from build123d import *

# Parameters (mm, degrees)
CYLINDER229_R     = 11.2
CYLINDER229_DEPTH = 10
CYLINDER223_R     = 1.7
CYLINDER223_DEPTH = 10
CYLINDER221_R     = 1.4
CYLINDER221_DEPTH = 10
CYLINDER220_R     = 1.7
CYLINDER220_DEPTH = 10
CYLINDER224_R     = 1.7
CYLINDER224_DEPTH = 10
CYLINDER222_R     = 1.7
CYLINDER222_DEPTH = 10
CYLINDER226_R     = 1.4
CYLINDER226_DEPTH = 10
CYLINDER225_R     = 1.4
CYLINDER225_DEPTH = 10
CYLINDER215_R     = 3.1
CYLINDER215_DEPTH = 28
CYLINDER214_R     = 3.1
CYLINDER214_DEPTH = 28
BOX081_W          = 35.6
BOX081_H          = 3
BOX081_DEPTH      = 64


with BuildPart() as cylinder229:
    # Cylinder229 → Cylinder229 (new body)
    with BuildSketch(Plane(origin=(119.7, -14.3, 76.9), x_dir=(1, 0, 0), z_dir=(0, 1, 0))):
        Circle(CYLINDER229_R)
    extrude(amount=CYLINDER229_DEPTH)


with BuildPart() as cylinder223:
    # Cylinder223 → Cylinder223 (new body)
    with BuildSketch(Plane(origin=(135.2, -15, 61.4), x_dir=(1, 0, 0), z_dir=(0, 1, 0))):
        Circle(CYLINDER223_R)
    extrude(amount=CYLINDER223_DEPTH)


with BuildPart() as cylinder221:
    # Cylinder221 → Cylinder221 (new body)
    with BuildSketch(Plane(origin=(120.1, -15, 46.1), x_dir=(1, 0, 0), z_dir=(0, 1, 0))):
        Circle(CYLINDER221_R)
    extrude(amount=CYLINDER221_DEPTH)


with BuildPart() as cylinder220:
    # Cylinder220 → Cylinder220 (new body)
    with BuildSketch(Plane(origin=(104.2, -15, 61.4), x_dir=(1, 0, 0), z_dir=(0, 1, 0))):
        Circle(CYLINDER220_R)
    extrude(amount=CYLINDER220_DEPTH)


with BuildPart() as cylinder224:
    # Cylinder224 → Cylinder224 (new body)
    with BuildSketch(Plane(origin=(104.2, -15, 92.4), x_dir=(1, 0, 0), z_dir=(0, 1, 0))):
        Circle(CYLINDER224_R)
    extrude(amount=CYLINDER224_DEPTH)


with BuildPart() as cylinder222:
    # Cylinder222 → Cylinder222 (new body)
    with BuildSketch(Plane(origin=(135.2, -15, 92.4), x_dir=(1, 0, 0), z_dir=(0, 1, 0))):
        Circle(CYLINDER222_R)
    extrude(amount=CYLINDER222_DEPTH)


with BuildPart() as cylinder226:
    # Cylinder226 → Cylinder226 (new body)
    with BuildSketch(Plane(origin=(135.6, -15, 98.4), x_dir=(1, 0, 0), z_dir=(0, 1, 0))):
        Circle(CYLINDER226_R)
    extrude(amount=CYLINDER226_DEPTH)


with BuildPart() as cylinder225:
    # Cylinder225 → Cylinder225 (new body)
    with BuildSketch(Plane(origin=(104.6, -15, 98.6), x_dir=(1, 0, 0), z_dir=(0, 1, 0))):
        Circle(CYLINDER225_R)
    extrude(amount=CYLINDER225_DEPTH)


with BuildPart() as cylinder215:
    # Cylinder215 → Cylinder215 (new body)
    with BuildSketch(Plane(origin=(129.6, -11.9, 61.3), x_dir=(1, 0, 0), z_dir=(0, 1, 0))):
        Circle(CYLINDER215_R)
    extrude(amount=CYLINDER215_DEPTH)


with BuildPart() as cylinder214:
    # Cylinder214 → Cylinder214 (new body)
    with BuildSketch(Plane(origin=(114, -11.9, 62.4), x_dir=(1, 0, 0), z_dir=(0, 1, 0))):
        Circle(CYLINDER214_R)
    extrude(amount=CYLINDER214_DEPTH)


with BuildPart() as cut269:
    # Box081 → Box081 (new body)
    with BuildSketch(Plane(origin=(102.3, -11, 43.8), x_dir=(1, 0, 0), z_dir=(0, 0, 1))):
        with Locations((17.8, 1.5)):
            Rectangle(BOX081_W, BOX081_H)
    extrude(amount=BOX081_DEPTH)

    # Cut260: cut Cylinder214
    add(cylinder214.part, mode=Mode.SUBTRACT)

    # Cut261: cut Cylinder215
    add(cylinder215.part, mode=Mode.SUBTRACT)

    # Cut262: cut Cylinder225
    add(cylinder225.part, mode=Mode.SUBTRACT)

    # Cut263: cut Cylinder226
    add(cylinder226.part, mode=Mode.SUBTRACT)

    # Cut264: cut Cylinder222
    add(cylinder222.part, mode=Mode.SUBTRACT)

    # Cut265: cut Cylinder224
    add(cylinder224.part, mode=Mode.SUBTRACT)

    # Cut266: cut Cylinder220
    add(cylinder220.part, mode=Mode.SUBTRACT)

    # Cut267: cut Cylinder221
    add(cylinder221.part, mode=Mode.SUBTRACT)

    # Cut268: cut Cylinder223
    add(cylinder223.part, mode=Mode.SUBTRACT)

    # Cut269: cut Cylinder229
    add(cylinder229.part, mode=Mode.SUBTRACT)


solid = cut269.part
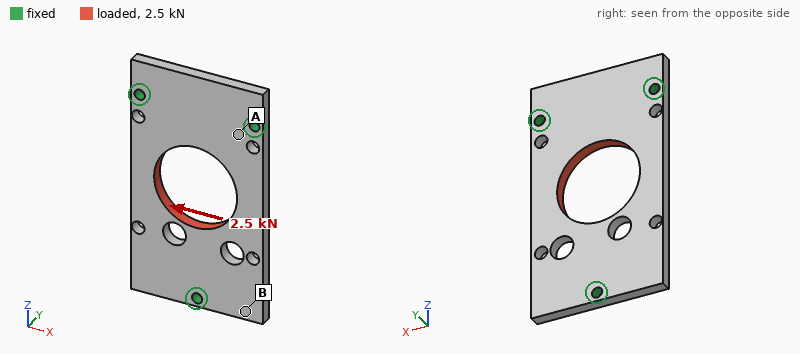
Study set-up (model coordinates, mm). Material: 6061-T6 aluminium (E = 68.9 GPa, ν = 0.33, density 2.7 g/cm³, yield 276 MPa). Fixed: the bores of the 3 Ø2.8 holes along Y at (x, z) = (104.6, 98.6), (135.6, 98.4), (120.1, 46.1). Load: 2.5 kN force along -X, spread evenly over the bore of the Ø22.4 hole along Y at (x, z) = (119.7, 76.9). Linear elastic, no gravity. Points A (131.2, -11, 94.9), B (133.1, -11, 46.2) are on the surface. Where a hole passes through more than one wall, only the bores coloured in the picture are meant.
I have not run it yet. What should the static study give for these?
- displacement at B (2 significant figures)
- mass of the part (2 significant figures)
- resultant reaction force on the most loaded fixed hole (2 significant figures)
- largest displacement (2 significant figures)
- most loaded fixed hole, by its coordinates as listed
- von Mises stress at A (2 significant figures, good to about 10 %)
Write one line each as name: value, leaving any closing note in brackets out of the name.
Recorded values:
displacement at B: 12 µm
mass of the part: 14 g
resultant reaction force on the most loaded fixed hole: 940 N
largest displacement: 33 µm
most loaded fixed hole, by its coordinates as listed: (120.1, 46.1)
von Mises stress at A: 33 MPa
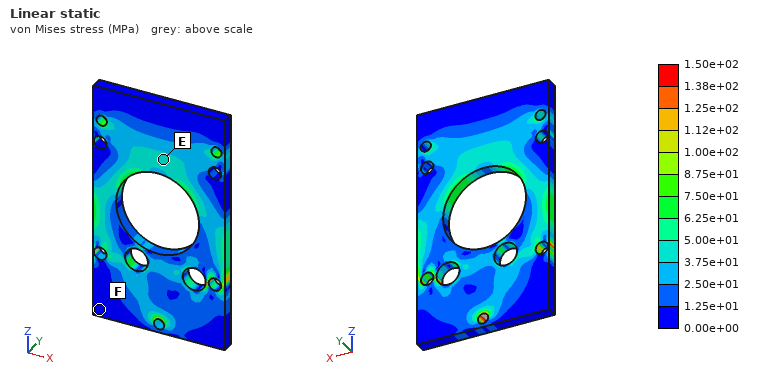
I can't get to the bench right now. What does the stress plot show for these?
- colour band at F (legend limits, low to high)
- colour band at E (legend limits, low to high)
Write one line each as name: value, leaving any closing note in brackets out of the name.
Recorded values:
colour band at F: 0.00e+00 to 1.25e+01 MPa
colour band at E: 3.75e+01 to 5.00e+01 MPa
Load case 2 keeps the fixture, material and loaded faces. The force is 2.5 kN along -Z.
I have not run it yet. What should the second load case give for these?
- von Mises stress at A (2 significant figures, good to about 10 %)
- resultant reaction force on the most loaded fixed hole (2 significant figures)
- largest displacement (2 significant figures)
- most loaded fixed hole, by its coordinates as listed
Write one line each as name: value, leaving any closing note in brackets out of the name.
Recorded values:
von Mises stress at A: 23 MPa
resultant reaction force on the most loaded fixed hole: 910 N
largest displacement: 13 µm
most loaded fixed hole, by its coordinates as listed: (120.1, 46.1)
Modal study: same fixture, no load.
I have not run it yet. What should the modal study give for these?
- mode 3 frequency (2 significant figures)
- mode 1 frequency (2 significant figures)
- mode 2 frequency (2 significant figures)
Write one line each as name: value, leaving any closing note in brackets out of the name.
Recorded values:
mode 3 frequency: 9200 Hz
mode 1 frequency: 4700 Hz
mode 2 frequency: 4800 Hz
